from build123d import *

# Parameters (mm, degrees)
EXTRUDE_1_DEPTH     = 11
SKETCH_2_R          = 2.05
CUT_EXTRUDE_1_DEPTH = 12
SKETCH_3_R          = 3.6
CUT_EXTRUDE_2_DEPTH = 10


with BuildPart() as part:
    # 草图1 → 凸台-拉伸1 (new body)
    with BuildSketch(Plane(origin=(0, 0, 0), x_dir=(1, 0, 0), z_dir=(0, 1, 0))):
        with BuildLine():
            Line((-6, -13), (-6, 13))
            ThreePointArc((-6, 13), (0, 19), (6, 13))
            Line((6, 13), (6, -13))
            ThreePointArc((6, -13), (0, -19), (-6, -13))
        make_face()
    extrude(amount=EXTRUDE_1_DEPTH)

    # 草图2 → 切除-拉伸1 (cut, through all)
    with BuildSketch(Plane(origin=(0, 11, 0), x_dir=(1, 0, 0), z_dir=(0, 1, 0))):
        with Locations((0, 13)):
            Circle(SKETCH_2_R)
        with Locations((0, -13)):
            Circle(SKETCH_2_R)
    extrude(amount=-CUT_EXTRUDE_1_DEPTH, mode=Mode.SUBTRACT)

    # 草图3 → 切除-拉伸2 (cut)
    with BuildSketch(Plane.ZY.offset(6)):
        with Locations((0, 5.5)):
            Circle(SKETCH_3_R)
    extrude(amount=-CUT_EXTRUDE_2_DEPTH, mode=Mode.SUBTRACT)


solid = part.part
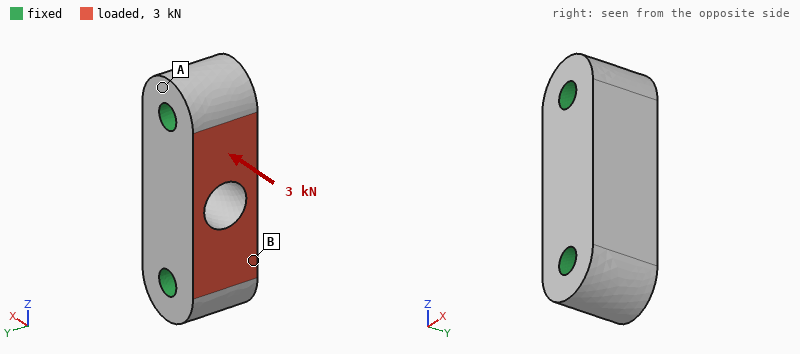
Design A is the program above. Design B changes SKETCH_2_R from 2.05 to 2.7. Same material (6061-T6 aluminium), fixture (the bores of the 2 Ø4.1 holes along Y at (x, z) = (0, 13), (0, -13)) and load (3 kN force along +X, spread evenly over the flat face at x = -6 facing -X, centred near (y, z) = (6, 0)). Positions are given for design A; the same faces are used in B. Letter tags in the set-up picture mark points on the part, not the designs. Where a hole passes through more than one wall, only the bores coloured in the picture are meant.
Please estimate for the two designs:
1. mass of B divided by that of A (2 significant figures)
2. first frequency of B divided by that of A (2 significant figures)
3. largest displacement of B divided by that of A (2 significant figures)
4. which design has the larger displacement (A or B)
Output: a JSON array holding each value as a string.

["0.95", "1.2", "0.81", "A"]
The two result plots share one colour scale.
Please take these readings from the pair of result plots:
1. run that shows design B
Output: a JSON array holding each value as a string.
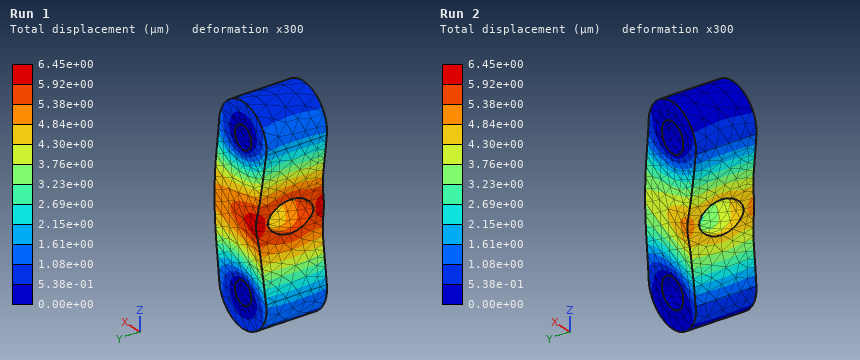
["Run 2"]
